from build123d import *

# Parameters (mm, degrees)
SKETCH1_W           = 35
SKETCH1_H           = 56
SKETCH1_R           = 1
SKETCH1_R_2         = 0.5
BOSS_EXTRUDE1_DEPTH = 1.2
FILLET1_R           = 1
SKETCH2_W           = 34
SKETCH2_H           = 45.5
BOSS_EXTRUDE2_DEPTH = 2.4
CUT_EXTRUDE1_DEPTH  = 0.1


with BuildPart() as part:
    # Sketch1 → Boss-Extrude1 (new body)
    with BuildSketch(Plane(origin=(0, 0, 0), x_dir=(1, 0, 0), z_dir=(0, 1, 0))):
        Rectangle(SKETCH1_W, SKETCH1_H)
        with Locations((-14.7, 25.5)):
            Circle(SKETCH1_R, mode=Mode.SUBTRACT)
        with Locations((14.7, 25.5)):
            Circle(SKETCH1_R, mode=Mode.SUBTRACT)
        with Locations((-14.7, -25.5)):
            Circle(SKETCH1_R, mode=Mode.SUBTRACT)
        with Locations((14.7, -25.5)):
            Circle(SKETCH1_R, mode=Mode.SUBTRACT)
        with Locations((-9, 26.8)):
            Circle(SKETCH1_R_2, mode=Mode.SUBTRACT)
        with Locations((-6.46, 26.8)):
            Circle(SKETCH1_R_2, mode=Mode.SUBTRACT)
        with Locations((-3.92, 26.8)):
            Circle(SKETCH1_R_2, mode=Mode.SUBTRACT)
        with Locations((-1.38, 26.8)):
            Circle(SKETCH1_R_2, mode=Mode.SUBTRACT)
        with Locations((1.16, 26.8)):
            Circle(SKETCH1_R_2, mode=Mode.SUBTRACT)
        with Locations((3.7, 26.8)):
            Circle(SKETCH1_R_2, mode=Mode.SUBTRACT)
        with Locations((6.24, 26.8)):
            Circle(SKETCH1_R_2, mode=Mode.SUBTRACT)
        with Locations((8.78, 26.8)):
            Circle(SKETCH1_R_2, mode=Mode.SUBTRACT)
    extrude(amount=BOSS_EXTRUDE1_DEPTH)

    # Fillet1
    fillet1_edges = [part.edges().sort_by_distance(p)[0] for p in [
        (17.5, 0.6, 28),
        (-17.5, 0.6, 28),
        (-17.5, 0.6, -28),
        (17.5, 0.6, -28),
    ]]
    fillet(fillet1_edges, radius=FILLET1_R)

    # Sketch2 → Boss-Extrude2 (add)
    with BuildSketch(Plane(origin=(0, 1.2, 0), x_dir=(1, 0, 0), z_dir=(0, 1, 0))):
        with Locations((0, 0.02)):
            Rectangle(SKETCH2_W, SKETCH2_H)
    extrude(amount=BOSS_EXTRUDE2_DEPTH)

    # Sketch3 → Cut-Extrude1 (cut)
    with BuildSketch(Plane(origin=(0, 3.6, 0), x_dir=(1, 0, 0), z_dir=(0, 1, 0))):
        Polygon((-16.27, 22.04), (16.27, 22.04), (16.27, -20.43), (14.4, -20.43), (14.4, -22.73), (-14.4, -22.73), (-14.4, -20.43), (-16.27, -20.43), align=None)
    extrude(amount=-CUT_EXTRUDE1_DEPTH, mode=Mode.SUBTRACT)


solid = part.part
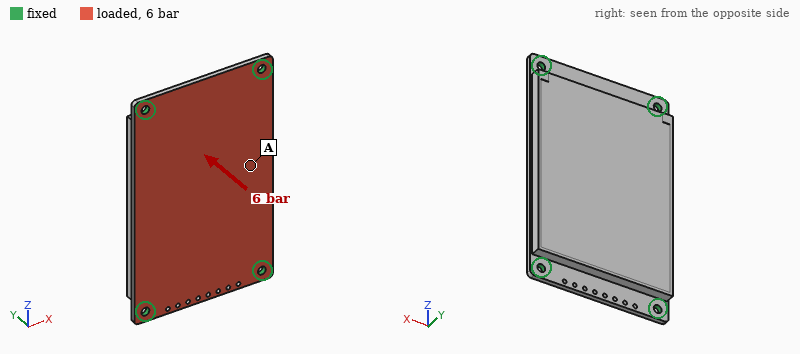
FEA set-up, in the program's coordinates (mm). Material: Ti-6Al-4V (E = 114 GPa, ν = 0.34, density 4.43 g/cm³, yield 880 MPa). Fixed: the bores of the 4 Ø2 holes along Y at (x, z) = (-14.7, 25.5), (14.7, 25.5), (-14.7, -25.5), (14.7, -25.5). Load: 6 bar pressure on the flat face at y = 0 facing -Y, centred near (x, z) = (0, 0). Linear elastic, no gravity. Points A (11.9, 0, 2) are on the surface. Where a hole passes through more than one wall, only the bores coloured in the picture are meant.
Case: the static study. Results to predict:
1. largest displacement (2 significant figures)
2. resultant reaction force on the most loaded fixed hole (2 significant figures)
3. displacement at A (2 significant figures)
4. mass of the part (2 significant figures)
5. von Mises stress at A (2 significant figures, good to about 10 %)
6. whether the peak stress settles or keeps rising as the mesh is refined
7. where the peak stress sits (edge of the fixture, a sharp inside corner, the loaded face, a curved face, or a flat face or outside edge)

77 µm
650 N
74 µm
26 g
47 MPa
keeps rising
edge of the fixture
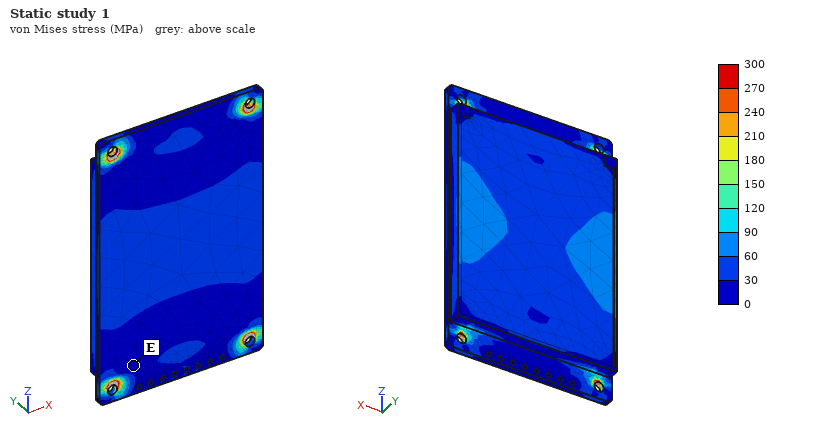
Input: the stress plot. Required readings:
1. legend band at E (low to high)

0 to 30 MPa
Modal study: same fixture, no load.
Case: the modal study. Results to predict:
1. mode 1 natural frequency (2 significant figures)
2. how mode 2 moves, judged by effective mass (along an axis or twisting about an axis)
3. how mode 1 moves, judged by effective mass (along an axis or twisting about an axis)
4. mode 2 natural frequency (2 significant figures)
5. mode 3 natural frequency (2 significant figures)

4100 Hz
twisting about Z
along Y
7100 Hz
10 kHz
